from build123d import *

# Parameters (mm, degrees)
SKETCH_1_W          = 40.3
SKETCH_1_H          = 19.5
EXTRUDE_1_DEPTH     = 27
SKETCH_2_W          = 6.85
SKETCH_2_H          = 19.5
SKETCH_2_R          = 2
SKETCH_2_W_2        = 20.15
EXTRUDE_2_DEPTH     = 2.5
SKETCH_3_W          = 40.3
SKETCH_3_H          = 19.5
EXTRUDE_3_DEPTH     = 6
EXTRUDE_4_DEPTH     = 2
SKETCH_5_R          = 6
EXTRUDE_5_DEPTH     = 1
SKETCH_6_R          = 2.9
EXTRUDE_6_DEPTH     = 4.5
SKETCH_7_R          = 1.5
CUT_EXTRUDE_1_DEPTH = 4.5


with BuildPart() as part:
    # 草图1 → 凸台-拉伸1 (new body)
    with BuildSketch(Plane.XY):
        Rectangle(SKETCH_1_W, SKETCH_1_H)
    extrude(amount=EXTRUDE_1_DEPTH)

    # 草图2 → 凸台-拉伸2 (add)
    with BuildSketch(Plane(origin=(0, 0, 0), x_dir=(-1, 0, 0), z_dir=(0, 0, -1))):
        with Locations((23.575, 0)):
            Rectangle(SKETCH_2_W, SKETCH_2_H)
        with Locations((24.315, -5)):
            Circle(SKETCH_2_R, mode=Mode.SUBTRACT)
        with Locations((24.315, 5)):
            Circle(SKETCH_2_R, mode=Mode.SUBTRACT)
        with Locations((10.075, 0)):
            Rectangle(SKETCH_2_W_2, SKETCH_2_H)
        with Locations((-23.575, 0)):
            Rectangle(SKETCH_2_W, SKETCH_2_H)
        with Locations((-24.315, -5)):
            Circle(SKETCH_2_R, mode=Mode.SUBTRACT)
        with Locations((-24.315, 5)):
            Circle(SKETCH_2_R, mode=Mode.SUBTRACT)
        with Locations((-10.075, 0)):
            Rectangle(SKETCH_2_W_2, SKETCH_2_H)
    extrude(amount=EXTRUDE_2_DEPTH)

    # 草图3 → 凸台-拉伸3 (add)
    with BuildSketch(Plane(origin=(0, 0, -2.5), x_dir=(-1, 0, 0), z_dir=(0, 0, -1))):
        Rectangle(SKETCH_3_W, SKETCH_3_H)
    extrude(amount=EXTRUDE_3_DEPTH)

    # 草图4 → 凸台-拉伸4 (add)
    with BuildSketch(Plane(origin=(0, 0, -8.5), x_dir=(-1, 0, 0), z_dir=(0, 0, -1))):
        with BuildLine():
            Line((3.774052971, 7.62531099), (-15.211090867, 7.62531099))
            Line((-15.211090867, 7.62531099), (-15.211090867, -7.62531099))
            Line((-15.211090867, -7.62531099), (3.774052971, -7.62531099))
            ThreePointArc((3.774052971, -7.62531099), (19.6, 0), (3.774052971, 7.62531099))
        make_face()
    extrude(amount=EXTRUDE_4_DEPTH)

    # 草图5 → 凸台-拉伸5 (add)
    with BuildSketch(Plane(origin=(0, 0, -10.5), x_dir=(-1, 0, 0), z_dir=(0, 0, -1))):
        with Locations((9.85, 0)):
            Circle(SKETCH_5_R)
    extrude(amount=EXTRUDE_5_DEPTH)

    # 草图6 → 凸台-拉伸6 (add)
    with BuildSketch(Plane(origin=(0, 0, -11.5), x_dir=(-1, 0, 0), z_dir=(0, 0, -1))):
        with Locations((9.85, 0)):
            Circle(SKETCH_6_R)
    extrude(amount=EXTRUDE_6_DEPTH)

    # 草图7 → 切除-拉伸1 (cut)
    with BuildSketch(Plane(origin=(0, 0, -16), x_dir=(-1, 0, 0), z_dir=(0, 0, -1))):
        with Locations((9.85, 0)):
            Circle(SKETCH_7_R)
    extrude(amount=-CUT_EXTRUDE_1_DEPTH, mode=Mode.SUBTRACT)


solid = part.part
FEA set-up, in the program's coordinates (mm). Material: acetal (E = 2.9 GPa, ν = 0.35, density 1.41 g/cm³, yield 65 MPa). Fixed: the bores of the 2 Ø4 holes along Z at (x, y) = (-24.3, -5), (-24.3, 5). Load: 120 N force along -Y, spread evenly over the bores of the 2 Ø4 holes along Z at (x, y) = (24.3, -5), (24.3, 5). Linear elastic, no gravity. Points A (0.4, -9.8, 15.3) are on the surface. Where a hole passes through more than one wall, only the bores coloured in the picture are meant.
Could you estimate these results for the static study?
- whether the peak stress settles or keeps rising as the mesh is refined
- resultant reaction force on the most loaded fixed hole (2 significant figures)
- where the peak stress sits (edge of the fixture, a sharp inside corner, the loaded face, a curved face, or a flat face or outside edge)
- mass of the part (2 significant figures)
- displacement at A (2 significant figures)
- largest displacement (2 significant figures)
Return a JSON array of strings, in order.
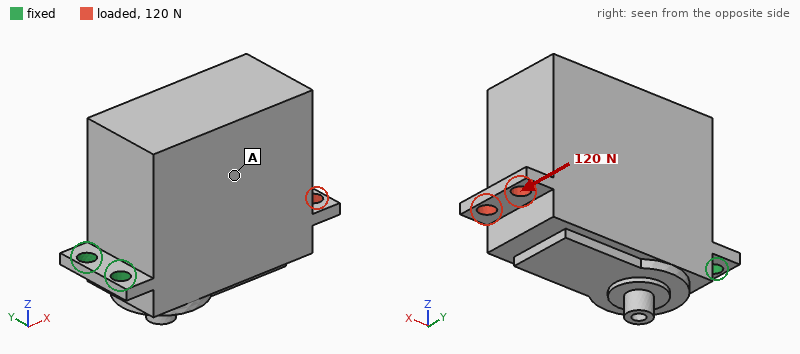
["keeps rising", "470 N", "edge of the fixture", "42 g", "0.23 mm", "0.56 mm"]
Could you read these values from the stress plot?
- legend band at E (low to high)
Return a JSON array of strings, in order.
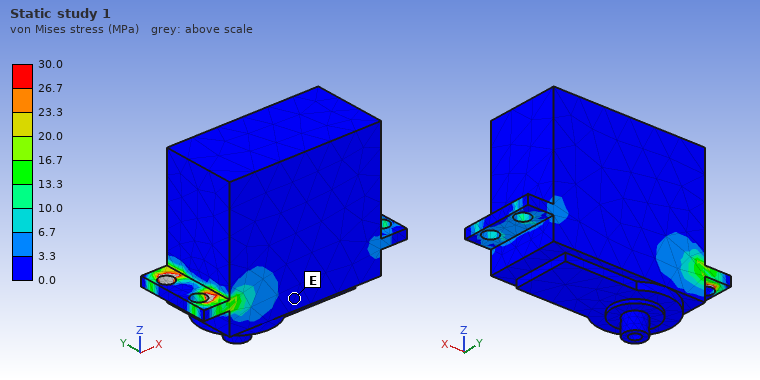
["0.0 to 3.3 MPa"]
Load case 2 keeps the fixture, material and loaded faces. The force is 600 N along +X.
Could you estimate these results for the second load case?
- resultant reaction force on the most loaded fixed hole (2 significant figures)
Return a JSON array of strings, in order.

["300 N"]
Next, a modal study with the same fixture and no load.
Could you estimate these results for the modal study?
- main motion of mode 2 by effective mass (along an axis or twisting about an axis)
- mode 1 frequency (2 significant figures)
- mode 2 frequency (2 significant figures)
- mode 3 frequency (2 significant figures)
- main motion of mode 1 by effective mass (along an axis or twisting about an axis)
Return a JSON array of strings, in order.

["along Y", "130 Hz", "580 Hz", "1000 Hz", "along Z"]
